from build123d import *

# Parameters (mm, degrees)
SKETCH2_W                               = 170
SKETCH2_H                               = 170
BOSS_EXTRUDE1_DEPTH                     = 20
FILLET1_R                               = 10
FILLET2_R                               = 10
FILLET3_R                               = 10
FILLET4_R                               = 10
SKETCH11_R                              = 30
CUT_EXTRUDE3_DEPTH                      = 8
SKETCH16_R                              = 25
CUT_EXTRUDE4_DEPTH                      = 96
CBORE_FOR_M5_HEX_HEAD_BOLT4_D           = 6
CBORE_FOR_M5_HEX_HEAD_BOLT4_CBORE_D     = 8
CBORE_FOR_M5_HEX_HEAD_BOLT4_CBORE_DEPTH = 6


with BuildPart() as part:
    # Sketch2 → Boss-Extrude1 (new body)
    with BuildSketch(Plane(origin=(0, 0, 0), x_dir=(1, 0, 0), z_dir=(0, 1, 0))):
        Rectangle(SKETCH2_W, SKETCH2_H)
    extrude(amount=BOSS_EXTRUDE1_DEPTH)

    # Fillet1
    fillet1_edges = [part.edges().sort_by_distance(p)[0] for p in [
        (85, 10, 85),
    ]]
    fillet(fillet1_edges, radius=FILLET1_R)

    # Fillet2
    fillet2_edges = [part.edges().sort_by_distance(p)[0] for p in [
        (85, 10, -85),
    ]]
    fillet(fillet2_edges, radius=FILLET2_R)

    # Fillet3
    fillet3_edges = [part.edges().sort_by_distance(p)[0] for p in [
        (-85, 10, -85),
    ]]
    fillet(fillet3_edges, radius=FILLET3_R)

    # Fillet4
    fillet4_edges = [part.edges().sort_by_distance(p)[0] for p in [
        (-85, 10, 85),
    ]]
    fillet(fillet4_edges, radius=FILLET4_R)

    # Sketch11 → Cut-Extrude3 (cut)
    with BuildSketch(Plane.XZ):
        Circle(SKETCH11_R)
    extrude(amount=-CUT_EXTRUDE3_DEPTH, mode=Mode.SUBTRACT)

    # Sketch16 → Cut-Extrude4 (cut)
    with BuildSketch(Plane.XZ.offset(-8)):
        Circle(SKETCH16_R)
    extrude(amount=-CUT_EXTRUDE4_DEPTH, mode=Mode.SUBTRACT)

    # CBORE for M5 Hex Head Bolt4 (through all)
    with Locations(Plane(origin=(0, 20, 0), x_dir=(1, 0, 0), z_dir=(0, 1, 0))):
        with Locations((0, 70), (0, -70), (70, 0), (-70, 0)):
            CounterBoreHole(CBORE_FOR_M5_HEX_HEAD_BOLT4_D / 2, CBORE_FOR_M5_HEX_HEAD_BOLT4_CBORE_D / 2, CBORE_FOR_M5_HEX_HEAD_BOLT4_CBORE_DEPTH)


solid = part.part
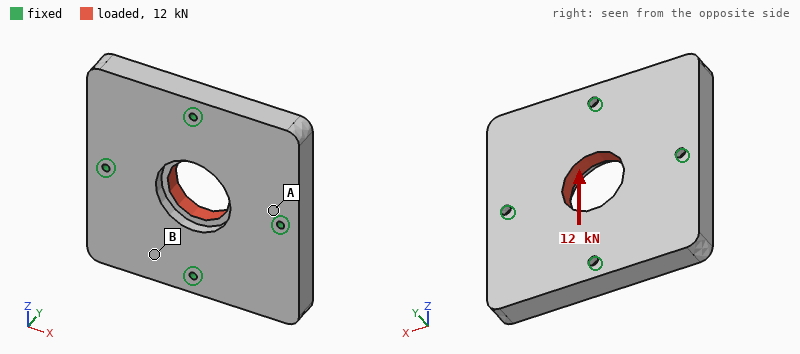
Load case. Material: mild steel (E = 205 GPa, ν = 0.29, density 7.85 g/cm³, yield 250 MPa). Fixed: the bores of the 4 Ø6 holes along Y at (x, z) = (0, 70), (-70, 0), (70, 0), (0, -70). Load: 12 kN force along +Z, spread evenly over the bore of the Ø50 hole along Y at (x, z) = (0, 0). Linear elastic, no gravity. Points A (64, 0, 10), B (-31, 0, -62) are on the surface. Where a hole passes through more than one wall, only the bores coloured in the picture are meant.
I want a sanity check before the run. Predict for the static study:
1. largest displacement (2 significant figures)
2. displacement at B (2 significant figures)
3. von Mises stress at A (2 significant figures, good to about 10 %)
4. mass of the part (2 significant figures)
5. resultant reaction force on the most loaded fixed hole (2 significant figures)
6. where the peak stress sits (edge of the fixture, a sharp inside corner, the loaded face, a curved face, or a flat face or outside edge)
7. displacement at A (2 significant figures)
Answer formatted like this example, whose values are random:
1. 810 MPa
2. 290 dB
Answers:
1. 1.9 µm
2. 0.79 µm
3. 4.0 MPa
4. 4.1 kg
5. 3.5 kN
6. edge of the fixture
7. 0.30 µm
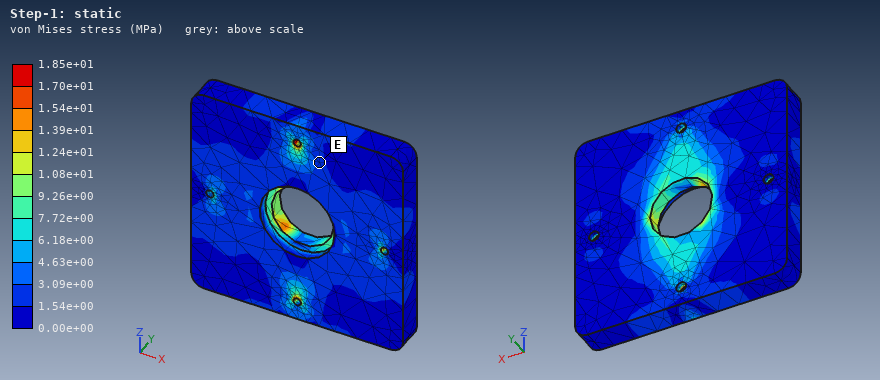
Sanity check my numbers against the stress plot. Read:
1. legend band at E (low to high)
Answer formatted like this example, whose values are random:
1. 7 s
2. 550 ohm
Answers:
1. 1.54e+00 to 3.09e+00 MPa
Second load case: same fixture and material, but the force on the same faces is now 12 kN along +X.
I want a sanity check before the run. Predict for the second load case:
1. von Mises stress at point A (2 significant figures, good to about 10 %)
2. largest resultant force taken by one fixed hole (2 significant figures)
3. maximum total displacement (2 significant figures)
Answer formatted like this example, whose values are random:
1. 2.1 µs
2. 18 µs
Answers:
1. 3.5 MPa
2. 3.5 kN
3. 1.9 µm
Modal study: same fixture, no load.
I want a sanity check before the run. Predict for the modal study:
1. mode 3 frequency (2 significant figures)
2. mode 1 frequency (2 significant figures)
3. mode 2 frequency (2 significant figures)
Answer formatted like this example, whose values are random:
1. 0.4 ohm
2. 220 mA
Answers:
1. 3500 Hz
2. 2900 Hz
3. 3500 Hz
